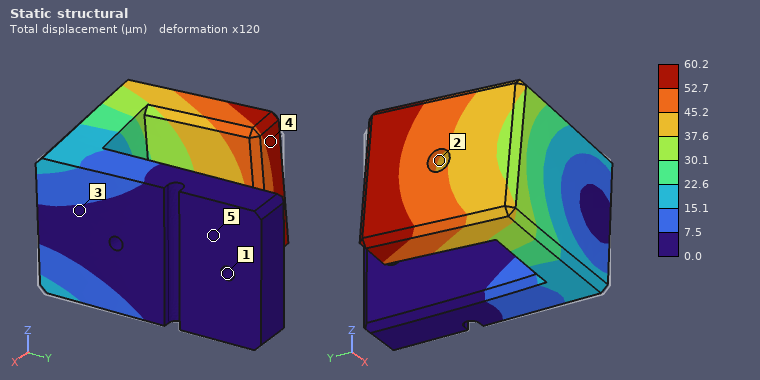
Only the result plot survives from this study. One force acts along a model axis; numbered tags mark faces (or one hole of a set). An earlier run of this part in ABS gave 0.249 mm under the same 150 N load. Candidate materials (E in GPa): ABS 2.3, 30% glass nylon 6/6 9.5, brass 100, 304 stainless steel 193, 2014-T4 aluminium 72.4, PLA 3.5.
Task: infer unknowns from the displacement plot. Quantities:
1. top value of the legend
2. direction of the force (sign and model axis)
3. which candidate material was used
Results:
60.2 µm
+Z
30% glass nylon 6/6
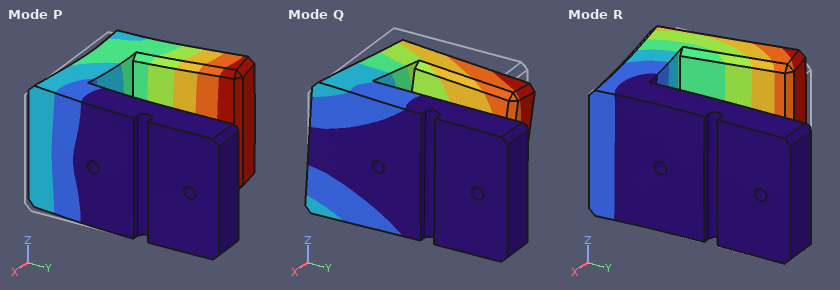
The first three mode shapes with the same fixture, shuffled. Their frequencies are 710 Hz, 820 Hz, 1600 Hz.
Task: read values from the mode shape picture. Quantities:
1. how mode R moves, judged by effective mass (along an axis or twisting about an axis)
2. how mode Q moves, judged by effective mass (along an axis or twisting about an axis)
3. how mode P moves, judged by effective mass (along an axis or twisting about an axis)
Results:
along Y
along Z
along X
